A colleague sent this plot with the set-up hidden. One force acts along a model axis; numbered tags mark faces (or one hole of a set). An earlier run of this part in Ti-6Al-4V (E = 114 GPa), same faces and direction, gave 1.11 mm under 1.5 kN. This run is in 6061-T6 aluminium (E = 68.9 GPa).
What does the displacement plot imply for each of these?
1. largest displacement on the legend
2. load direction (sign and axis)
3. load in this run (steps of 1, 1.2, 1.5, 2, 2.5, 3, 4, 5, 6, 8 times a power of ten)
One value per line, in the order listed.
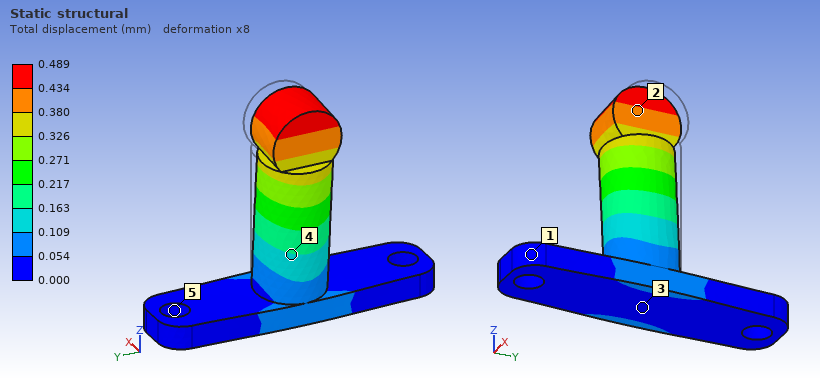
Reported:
0.489 mm
-X
400 N
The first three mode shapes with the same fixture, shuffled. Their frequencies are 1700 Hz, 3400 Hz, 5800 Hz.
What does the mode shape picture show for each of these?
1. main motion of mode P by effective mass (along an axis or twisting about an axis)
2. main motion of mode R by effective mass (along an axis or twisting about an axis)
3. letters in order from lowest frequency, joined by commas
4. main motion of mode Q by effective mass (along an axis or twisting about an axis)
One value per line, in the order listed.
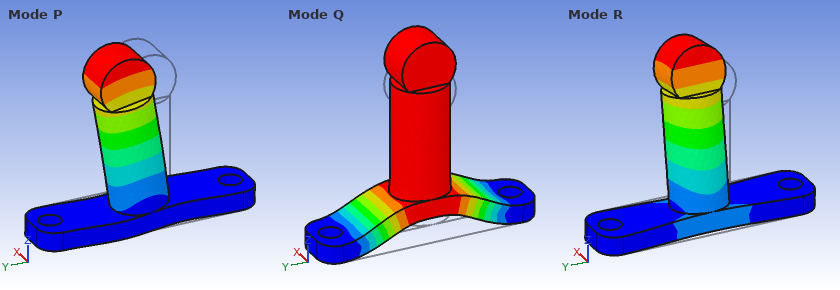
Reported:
along Y
along X
R, P, Q
along Z
